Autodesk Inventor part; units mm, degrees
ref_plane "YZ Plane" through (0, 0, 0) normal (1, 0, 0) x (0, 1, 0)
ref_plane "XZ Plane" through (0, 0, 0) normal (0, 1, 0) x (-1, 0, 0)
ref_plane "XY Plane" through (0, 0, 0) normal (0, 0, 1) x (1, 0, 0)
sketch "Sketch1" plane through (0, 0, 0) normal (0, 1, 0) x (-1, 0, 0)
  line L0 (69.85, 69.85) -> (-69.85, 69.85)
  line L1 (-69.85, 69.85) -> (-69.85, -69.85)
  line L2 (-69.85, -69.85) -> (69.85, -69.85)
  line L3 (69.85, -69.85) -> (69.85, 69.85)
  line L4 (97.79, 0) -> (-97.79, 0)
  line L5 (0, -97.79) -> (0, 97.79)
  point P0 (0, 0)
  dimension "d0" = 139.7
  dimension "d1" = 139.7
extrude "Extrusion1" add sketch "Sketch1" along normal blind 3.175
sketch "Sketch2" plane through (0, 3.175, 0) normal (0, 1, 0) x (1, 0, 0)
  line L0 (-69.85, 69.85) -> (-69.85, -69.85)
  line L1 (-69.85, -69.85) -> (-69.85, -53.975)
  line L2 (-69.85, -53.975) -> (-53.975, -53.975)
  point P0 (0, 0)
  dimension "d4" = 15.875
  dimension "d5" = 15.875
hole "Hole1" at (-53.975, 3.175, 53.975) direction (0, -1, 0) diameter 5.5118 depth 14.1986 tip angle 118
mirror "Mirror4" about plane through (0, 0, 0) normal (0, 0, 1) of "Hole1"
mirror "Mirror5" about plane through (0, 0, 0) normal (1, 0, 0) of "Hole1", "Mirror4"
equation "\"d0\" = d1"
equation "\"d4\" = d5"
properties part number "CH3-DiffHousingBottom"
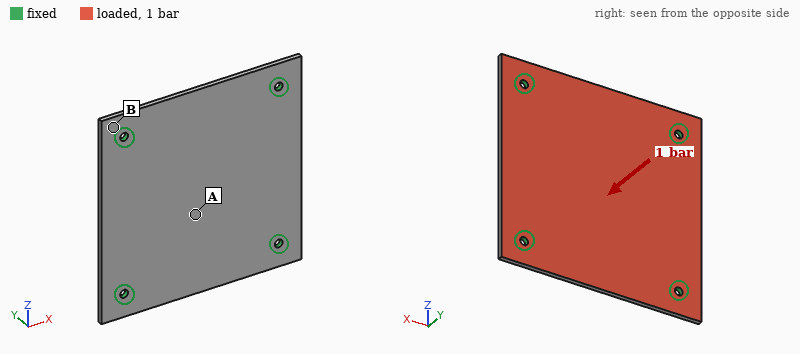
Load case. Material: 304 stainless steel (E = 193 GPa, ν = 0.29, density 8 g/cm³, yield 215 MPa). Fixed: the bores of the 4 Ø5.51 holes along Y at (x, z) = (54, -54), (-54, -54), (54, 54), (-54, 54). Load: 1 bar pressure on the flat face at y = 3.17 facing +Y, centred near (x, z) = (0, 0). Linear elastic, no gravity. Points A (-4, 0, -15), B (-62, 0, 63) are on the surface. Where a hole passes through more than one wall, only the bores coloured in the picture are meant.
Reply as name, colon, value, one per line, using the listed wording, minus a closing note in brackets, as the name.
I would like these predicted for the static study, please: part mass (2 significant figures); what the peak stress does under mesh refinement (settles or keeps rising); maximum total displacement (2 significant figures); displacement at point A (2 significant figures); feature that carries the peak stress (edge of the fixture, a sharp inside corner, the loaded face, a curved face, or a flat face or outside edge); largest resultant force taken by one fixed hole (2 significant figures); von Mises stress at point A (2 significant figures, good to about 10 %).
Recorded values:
part mass: 490 g
what the peak stress does under mesh refinement: keeps rising
maximum total displacement: 0.17 mm
displacement at point A: 0.16 mm
feature that carries the peak stress: edge of the fixture
largest resultant force taken by one fixed hole: 490 N
von Mises stress at point A: 33 MPa
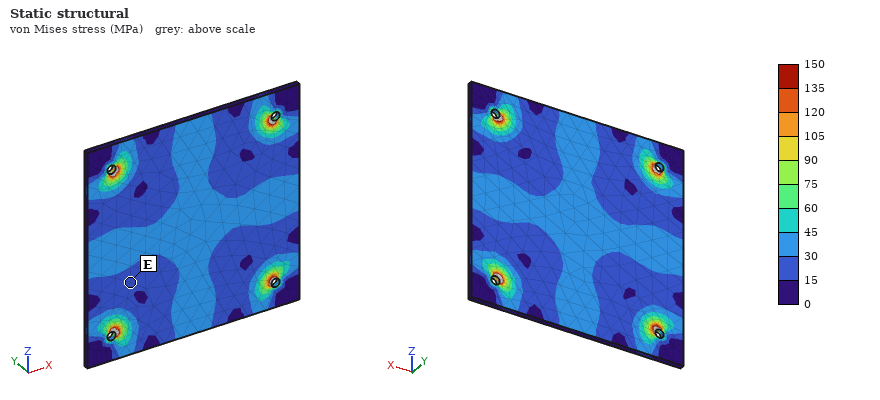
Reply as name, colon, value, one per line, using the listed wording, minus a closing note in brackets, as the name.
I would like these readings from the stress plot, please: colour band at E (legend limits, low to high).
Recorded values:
colour band at E: 15 to 30 MPa
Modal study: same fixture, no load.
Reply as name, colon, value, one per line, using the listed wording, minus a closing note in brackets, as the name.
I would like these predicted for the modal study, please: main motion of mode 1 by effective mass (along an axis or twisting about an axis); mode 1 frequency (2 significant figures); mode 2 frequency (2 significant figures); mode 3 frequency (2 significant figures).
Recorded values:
main motion of mode 1 by effective mass: along Y
mode 1 frequency: 930 Hz
mode 2 frequency: 1500 Hz
mode 3 frequency: 1500 Hz
